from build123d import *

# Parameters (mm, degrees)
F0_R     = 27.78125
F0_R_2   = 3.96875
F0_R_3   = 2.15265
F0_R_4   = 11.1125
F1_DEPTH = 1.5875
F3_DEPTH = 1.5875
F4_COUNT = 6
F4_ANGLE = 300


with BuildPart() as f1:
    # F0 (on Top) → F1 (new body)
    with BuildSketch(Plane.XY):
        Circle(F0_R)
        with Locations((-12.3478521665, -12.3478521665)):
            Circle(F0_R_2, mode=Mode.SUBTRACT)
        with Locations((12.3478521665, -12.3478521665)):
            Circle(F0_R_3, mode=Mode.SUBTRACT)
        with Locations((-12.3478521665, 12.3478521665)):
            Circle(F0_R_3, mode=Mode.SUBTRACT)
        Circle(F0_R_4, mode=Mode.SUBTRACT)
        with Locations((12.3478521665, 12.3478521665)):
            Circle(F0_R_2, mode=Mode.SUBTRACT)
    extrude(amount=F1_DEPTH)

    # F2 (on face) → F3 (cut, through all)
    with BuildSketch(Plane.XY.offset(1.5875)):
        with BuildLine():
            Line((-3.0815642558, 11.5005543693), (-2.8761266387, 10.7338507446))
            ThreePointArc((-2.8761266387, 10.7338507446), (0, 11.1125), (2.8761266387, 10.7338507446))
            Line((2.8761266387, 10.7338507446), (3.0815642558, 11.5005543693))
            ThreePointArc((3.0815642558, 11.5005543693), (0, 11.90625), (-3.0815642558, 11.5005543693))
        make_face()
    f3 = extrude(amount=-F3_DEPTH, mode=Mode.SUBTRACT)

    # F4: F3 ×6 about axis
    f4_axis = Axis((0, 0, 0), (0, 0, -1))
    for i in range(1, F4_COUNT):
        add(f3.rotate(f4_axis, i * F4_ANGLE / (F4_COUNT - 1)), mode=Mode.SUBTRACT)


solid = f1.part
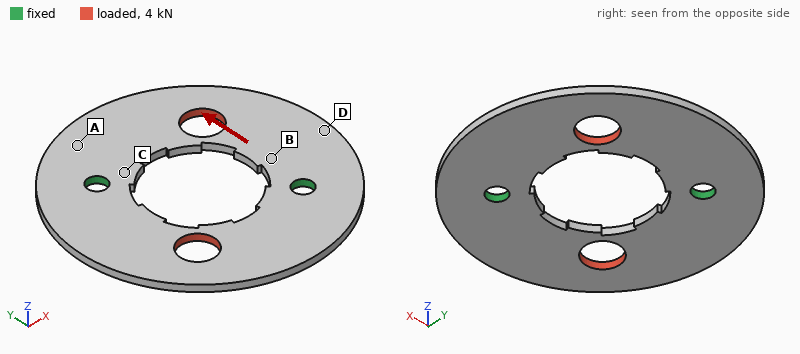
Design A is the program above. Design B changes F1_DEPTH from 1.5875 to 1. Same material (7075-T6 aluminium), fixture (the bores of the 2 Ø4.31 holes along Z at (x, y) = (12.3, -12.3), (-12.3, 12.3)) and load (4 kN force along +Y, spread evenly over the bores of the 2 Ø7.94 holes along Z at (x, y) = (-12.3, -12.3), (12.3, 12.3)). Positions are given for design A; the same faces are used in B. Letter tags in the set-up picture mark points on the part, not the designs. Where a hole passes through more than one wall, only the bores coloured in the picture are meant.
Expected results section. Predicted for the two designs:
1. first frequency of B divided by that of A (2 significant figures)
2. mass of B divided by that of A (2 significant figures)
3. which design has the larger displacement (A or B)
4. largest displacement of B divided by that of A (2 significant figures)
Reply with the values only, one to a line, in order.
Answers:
0.64
0.63
B
1.6
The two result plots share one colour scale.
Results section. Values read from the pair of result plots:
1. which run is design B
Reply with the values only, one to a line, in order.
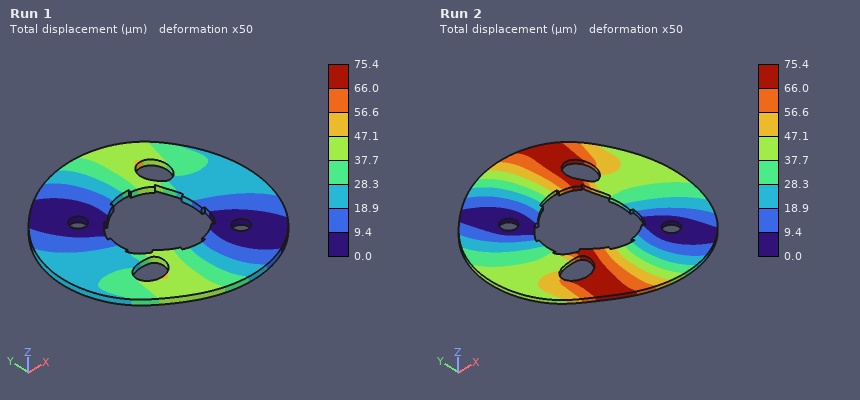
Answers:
Run 2
